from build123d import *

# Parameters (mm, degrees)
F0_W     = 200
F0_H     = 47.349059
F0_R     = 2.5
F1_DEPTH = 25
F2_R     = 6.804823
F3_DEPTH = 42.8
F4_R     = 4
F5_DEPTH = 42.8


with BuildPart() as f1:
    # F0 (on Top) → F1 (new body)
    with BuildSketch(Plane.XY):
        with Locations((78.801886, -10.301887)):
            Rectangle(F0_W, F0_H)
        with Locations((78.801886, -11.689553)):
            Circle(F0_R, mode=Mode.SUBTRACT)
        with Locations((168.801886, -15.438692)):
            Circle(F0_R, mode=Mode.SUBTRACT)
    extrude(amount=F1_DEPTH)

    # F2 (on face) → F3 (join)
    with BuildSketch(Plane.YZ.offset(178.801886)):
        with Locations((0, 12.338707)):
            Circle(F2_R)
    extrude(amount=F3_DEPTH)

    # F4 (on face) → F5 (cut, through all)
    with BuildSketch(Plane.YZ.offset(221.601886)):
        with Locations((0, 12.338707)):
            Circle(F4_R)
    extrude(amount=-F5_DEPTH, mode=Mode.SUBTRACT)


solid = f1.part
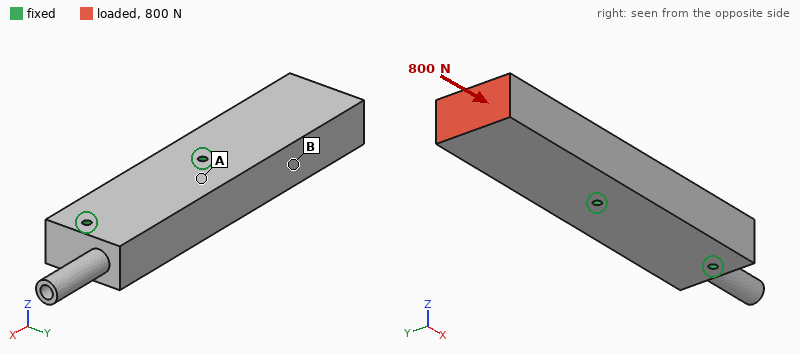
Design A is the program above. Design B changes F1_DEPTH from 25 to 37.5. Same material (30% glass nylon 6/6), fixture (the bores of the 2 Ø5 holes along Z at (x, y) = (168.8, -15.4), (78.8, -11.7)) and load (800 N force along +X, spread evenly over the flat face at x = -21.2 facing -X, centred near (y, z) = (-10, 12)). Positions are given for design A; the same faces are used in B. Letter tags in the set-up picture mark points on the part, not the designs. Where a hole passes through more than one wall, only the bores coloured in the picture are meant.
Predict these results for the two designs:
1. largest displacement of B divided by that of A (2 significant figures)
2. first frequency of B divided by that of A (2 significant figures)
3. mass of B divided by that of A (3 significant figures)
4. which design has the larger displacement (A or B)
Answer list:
0.67
1.3
1.49
A
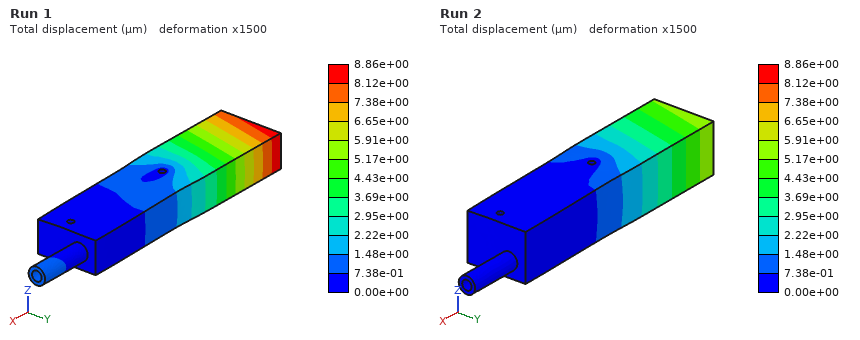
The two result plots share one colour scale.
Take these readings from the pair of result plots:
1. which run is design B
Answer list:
Run 2
